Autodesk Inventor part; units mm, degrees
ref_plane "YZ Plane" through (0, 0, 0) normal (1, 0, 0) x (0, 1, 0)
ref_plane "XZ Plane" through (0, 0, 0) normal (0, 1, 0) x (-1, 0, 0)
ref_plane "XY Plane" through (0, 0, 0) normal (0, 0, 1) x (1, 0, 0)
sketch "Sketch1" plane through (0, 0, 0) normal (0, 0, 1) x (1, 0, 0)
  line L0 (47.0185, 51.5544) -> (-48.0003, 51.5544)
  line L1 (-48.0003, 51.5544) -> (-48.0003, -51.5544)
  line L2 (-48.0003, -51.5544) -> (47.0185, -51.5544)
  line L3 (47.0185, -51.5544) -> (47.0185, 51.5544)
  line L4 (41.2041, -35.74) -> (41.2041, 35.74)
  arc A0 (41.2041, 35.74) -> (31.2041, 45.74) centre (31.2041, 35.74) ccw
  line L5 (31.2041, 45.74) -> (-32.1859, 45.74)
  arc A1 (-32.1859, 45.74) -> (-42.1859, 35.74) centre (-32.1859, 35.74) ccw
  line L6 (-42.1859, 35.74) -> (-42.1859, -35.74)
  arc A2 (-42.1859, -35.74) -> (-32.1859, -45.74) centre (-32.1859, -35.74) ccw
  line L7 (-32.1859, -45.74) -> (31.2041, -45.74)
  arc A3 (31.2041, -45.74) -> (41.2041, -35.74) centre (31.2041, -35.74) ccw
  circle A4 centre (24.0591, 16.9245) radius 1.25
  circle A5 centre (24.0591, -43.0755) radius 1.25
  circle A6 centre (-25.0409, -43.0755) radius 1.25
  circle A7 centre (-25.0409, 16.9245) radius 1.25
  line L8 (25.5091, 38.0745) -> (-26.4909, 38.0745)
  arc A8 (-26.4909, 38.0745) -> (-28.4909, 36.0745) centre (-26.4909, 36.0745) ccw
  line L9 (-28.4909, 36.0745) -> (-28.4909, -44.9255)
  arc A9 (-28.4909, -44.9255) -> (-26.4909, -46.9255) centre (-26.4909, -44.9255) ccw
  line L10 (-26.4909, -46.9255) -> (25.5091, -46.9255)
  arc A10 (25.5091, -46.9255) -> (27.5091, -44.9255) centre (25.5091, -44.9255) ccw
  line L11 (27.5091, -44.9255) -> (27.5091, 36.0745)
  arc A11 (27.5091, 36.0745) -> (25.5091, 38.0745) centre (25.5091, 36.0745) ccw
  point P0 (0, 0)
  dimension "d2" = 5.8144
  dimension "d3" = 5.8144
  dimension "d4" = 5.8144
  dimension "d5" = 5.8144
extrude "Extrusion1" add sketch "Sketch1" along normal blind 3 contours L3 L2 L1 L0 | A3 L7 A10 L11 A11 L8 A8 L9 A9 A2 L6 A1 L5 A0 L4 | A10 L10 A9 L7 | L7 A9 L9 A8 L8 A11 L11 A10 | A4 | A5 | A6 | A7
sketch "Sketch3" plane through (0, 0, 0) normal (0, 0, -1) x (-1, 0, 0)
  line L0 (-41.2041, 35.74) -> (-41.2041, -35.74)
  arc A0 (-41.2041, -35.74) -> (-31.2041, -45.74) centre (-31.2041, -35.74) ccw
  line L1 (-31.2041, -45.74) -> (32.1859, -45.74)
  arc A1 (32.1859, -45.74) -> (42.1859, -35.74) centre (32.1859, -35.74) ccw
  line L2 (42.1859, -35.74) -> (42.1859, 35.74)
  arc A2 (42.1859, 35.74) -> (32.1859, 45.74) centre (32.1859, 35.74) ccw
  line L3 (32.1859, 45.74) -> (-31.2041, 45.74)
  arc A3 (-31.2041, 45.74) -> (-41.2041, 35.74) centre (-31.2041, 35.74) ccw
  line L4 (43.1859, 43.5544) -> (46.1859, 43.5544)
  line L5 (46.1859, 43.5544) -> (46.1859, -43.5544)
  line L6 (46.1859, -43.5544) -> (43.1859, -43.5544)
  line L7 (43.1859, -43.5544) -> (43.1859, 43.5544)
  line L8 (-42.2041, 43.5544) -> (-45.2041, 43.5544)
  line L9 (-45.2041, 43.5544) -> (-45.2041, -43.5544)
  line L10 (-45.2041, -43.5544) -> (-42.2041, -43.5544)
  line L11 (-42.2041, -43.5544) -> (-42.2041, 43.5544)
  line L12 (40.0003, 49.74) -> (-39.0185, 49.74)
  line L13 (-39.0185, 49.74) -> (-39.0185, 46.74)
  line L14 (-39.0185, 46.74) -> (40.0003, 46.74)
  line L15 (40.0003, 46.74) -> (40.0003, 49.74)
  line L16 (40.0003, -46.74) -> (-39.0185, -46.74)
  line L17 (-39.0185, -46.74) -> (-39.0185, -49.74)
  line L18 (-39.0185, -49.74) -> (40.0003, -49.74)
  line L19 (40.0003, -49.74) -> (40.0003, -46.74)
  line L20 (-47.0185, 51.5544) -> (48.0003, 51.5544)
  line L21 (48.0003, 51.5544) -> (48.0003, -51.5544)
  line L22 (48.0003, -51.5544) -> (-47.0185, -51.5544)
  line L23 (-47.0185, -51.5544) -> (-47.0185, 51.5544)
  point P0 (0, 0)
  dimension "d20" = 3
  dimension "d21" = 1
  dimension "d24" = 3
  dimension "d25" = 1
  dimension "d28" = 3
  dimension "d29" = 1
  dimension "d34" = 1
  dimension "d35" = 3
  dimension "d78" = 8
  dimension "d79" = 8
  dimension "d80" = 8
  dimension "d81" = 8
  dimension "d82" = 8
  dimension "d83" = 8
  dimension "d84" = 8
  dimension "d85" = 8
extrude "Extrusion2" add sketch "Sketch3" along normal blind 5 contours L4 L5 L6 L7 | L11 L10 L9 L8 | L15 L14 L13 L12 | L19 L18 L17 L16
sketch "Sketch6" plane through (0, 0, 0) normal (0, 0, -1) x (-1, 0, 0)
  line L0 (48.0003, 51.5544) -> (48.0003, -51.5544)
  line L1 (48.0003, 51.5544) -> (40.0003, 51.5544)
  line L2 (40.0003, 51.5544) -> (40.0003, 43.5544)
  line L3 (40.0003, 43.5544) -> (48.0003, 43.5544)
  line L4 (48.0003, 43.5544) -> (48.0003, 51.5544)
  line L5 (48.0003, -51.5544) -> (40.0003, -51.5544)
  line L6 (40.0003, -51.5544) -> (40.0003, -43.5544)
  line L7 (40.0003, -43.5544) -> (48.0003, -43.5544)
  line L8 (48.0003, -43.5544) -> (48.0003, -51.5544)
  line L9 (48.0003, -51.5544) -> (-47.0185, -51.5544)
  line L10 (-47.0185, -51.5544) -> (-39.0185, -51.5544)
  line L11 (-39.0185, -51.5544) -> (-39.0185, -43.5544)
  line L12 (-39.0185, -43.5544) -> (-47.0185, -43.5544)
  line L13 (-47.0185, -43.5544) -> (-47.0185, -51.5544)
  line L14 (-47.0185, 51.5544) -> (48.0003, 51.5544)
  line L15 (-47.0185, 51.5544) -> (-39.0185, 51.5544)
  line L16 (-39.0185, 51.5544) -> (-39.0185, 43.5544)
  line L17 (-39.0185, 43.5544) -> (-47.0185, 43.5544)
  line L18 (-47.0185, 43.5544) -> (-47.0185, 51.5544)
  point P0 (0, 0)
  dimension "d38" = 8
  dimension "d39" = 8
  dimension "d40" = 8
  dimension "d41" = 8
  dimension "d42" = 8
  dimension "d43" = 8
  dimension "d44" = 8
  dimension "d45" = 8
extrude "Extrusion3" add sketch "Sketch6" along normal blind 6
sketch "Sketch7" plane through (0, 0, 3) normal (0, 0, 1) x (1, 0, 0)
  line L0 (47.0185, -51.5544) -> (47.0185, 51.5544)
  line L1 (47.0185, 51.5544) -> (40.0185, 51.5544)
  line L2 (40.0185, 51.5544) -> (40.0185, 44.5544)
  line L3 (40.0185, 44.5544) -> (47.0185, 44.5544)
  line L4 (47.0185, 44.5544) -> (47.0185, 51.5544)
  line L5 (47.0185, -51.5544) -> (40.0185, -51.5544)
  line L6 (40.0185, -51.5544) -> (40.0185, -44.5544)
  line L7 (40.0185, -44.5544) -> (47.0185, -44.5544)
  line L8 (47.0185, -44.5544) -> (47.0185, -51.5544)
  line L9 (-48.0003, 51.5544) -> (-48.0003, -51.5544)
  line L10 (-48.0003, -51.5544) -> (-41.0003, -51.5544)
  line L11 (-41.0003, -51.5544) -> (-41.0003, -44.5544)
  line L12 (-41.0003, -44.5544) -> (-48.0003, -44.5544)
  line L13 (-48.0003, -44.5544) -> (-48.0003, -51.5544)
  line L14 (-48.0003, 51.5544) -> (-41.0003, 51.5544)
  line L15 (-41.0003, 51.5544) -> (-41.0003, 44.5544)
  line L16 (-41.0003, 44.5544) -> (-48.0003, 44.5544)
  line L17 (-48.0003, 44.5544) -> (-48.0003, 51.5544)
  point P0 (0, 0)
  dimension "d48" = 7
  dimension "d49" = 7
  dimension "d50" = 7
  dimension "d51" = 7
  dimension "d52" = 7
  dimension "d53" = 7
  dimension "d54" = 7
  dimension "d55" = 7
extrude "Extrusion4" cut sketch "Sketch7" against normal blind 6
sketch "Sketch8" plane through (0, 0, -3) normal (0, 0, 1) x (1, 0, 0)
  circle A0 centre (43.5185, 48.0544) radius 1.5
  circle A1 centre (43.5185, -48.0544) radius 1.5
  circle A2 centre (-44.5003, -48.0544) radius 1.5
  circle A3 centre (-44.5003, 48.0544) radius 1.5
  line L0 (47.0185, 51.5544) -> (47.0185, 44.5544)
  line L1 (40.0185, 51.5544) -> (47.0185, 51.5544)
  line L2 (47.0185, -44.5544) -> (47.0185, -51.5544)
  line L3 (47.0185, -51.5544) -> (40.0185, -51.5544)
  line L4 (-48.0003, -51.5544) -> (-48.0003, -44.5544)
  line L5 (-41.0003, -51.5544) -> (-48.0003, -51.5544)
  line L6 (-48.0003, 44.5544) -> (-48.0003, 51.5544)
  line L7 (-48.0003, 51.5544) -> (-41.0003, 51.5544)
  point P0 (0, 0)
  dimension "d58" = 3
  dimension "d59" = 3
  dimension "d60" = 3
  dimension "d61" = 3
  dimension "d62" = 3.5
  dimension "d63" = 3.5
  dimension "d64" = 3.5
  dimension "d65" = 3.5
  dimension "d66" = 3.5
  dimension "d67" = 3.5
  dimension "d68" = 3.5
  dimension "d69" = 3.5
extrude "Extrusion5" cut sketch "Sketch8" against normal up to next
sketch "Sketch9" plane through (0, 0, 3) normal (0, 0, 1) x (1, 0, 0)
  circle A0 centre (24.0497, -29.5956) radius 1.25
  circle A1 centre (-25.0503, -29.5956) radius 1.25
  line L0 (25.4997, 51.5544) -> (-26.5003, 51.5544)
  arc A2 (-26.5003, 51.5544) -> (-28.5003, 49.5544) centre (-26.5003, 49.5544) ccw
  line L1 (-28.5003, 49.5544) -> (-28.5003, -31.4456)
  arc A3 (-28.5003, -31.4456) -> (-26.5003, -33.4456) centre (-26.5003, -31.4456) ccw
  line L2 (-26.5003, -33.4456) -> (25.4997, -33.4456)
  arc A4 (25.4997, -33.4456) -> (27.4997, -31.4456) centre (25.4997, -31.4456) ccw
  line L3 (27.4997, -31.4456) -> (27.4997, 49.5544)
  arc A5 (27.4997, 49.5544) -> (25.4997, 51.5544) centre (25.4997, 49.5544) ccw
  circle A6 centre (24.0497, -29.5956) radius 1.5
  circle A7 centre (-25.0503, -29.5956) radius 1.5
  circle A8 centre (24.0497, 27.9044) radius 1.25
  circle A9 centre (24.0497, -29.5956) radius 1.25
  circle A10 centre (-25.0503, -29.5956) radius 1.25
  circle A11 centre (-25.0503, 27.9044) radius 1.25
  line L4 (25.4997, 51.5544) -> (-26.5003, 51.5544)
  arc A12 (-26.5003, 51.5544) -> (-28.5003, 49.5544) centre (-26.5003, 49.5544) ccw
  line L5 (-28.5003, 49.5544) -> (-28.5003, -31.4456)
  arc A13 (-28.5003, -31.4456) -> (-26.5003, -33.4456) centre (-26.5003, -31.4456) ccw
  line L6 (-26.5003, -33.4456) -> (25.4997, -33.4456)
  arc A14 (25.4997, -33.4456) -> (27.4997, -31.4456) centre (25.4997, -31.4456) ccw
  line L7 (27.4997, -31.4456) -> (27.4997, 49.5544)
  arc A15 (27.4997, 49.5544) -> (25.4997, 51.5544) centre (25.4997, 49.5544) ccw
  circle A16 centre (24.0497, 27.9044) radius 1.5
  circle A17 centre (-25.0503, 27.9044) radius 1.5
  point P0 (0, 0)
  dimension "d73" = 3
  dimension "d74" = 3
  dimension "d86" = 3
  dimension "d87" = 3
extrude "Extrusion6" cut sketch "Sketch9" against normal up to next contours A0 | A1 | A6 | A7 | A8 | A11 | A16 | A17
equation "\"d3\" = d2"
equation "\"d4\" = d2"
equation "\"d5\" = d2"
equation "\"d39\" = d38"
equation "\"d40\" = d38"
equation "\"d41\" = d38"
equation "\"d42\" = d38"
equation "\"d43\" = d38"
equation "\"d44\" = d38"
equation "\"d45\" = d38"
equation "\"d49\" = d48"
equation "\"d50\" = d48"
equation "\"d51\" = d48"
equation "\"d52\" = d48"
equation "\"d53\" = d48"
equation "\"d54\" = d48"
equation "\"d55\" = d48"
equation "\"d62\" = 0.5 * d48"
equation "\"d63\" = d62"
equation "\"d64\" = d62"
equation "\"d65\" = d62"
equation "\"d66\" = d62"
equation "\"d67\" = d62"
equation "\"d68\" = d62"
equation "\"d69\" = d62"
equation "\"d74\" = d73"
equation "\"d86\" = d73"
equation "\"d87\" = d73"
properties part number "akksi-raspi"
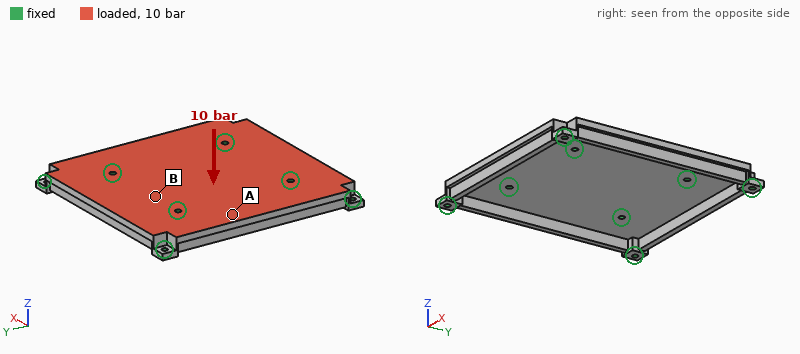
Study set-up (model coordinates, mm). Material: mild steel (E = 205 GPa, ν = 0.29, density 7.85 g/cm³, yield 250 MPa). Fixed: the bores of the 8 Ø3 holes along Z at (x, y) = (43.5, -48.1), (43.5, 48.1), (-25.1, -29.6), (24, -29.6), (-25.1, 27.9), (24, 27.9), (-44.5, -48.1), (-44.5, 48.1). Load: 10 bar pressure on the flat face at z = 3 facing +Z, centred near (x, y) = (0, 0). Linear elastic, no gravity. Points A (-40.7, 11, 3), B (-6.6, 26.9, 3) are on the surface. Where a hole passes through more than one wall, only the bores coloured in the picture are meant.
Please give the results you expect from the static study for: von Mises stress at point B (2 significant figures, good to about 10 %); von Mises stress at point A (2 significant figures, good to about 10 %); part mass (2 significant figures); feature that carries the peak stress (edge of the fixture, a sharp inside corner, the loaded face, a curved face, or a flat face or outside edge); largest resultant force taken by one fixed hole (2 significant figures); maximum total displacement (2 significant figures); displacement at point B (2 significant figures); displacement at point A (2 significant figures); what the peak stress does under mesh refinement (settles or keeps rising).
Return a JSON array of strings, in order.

["80 MPa", "49 MPa", "270 g", "edge of the fixture", "1.9 kN", "0.10 mm", "0.044 mm", "0.042 mm", "keeps rising"]
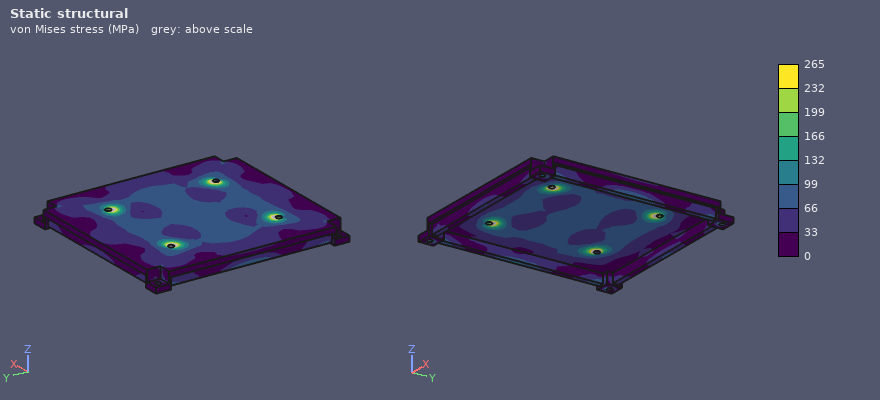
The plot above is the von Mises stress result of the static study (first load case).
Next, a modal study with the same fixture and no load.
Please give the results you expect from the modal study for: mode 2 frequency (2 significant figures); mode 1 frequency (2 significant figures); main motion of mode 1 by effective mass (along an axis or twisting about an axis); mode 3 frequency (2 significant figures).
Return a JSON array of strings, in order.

["4500 Hz", "3900 Hz", "along Z", "4500 Hz"]
